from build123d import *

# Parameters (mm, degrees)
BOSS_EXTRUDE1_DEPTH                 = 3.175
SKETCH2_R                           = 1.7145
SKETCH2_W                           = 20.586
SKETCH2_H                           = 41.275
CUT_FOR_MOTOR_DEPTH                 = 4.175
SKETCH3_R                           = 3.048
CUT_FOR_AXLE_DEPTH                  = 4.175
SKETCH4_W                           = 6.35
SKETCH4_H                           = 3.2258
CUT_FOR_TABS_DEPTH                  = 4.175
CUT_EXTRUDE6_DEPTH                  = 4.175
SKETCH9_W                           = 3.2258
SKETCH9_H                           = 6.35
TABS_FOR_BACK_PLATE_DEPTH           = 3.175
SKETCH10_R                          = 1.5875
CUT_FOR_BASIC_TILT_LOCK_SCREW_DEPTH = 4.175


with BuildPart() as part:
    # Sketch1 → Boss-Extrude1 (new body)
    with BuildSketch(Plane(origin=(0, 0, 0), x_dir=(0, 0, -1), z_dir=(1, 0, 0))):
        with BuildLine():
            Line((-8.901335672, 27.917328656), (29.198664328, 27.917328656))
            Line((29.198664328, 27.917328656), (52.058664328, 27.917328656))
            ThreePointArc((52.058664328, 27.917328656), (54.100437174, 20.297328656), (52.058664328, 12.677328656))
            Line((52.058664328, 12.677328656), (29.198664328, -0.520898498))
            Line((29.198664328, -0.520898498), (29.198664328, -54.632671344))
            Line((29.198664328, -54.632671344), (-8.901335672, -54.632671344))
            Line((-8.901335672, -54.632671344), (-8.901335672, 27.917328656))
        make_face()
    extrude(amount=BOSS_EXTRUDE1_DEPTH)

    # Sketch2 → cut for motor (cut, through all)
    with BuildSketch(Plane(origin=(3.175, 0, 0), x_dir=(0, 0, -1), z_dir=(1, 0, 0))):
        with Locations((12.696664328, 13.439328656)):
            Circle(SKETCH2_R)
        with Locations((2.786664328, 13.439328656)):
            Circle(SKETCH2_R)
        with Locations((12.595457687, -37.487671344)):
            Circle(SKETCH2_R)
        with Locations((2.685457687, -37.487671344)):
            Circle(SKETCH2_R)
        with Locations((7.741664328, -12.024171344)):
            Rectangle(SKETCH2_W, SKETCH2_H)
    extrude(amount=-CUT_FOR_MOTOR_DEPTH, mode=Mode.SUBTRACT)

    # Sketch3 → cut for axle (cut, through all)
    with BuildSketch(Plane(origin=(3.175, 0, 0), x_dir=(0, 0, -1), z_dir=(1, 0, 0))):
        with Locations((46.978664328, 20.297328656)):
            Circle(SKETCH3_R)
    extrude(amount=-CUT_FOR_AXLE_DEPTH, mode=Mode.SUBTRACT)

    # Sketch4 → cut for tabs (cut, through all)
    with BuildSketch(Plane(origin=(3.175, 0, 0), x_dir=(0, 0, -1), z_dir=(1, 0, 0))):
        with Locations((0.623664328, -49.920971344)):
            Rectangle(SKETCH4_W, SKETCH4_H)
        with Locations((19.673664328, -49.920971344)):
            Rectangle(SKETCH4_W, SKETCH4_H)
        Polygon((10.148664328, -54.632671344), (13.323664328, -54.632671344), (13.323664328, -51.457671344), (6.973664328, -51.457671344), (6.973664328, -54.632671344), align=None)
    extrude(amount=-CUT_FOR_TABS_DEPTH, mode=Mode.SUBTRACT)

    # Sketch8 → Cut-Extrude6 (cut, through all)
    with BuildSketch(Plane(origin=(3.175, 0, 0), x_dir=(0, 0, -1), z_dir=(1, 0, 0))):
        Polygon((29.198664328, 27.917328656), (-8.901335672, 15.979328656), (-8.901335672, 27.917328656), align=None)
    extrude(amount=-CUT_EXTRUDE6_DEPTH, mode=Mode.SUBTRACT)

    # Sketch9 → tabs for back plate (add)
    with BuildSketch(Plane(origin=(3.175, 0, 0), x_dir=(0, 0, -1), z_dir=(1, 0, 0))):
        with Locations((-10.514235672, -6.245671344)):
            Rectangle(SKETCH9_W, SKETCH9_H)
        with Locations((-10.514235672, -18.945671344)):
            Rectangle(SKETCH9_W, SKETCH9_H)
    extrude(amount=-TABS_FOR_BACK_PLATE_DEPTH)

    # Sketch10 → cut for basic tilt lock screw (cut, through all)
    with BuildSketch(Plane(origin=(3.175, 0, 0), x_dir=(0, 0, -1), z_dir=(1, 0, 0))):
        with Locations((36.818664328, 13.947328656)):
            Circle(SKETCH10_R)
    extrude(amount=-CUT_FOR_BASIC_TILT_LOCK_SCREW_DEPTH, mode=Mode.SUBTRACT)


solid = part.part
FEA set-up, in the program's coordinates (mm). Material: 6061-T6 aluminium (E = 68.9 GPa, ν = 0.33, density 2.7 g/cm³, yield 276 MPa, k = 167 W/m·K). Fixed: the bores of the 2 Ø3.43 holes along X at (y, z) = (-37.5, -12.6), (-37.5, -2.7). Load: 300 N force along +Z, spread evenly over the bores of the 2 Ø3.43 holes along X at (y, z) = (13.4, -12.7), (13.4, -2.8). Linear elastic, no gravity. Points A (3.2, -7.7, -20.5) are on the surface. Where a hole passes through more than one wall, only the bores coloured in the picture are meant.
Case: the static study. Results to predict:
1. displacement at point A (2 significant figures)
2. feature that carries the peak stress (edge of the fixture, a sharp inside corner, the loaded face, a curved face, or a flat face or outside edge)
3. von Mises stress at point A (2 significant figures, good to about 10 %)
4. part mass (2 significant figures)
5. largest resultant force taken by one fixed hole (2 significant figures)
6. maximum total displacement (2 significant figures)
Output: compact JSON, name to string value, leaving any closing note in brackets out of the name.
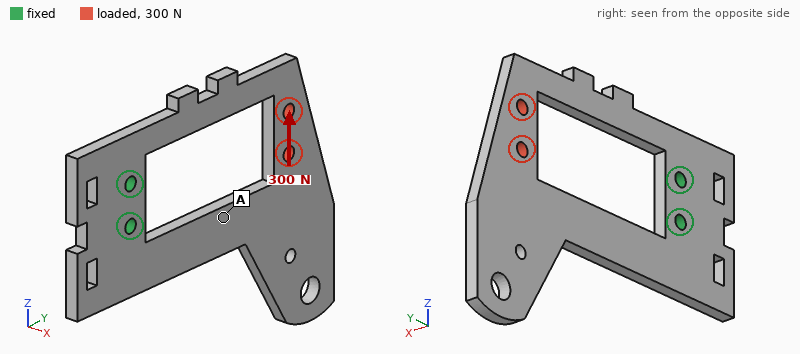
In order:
{"displacement at point A": "0.12 mm", "feature that carries the peak stress": "edge of the fixture", "von Mises stress at point A": "22 MPa", "part mass": "21 g", "largest resultant force taken by one fixed hole": "1.1 kN", "maximum total displacement": "0.27 mm"}
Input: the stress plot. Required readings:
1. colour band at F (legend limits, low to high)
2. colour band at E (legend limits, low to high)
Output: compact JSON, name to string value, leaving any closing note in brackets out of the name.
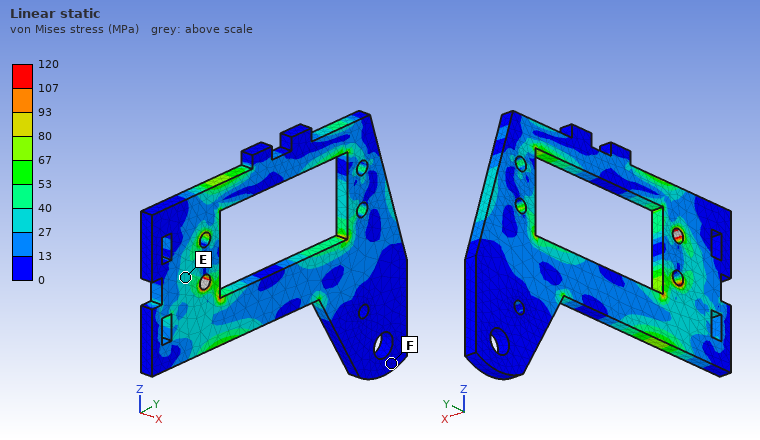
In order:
{"colour band at F": "0 to 13 MPa", "colour band at E": "27 to 40 MPa"}
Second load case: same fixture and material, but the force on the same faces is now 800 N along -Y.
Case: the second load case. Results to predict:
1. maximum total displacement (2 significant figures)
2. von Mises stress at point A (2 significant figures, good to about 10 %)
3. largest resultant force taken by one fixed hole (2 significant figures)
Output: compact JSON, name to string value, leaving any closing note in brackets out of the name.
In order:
{"maximum total displacement": "32 µm", "von Mises stress at point A": "19 MPa", "largest resultant force taken by one fixed hole": "440 N"}
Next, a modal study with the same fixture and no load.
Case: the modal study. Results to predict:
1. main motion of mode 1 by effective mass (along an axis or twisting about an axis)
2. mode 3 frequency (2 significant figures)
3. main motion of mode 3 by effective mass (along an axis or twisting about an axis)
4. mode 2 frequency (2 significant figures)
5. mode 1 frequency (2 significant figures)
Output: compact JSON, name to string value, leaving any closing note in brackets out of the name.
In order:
{"main motion of mode 1 by effective mass": "along X", "mode 3 frequency": "1800 Hz", "main motion of mode 3 by effective mass": "along Z", "mode 2 frequency": "1000 Hz", "mode 1 frequency": "360 Hz"}
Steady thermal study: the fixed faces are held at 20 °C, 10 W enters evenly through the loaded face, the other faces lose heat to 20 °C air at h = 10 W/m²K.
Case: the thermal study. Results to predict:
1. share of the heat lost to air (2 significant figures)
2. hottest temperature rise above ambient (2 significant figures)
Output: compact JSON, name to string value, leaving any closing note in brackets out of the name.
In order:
{"share of the heat lost to air": "17 %", "hottest temperature rise above ambient": "55 K"}
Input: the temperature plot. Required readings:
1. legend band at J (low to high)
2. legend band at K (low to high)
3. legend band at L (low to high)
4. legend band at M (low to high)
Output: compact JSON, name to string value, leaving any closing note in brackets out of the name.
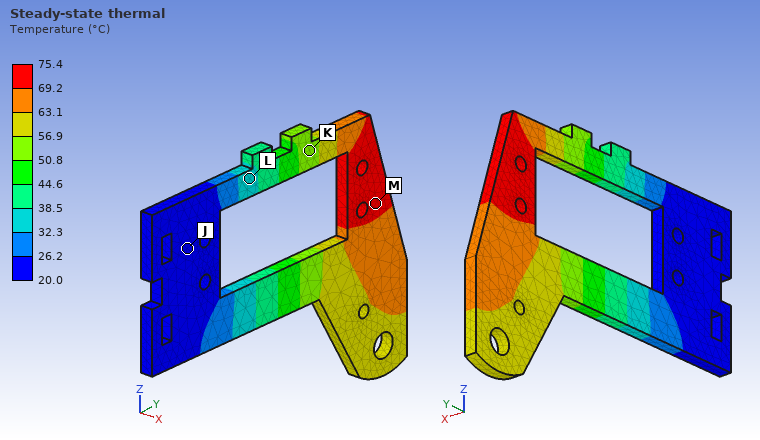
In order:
{"legend band at J": "20.0 to 26.2 °C", "legend band at K": "50.8 to 56.9 °C", "legend band at L": "32.3 to 38.5 °C", "legend band at M": "69.2 to 75.4 °C"}
